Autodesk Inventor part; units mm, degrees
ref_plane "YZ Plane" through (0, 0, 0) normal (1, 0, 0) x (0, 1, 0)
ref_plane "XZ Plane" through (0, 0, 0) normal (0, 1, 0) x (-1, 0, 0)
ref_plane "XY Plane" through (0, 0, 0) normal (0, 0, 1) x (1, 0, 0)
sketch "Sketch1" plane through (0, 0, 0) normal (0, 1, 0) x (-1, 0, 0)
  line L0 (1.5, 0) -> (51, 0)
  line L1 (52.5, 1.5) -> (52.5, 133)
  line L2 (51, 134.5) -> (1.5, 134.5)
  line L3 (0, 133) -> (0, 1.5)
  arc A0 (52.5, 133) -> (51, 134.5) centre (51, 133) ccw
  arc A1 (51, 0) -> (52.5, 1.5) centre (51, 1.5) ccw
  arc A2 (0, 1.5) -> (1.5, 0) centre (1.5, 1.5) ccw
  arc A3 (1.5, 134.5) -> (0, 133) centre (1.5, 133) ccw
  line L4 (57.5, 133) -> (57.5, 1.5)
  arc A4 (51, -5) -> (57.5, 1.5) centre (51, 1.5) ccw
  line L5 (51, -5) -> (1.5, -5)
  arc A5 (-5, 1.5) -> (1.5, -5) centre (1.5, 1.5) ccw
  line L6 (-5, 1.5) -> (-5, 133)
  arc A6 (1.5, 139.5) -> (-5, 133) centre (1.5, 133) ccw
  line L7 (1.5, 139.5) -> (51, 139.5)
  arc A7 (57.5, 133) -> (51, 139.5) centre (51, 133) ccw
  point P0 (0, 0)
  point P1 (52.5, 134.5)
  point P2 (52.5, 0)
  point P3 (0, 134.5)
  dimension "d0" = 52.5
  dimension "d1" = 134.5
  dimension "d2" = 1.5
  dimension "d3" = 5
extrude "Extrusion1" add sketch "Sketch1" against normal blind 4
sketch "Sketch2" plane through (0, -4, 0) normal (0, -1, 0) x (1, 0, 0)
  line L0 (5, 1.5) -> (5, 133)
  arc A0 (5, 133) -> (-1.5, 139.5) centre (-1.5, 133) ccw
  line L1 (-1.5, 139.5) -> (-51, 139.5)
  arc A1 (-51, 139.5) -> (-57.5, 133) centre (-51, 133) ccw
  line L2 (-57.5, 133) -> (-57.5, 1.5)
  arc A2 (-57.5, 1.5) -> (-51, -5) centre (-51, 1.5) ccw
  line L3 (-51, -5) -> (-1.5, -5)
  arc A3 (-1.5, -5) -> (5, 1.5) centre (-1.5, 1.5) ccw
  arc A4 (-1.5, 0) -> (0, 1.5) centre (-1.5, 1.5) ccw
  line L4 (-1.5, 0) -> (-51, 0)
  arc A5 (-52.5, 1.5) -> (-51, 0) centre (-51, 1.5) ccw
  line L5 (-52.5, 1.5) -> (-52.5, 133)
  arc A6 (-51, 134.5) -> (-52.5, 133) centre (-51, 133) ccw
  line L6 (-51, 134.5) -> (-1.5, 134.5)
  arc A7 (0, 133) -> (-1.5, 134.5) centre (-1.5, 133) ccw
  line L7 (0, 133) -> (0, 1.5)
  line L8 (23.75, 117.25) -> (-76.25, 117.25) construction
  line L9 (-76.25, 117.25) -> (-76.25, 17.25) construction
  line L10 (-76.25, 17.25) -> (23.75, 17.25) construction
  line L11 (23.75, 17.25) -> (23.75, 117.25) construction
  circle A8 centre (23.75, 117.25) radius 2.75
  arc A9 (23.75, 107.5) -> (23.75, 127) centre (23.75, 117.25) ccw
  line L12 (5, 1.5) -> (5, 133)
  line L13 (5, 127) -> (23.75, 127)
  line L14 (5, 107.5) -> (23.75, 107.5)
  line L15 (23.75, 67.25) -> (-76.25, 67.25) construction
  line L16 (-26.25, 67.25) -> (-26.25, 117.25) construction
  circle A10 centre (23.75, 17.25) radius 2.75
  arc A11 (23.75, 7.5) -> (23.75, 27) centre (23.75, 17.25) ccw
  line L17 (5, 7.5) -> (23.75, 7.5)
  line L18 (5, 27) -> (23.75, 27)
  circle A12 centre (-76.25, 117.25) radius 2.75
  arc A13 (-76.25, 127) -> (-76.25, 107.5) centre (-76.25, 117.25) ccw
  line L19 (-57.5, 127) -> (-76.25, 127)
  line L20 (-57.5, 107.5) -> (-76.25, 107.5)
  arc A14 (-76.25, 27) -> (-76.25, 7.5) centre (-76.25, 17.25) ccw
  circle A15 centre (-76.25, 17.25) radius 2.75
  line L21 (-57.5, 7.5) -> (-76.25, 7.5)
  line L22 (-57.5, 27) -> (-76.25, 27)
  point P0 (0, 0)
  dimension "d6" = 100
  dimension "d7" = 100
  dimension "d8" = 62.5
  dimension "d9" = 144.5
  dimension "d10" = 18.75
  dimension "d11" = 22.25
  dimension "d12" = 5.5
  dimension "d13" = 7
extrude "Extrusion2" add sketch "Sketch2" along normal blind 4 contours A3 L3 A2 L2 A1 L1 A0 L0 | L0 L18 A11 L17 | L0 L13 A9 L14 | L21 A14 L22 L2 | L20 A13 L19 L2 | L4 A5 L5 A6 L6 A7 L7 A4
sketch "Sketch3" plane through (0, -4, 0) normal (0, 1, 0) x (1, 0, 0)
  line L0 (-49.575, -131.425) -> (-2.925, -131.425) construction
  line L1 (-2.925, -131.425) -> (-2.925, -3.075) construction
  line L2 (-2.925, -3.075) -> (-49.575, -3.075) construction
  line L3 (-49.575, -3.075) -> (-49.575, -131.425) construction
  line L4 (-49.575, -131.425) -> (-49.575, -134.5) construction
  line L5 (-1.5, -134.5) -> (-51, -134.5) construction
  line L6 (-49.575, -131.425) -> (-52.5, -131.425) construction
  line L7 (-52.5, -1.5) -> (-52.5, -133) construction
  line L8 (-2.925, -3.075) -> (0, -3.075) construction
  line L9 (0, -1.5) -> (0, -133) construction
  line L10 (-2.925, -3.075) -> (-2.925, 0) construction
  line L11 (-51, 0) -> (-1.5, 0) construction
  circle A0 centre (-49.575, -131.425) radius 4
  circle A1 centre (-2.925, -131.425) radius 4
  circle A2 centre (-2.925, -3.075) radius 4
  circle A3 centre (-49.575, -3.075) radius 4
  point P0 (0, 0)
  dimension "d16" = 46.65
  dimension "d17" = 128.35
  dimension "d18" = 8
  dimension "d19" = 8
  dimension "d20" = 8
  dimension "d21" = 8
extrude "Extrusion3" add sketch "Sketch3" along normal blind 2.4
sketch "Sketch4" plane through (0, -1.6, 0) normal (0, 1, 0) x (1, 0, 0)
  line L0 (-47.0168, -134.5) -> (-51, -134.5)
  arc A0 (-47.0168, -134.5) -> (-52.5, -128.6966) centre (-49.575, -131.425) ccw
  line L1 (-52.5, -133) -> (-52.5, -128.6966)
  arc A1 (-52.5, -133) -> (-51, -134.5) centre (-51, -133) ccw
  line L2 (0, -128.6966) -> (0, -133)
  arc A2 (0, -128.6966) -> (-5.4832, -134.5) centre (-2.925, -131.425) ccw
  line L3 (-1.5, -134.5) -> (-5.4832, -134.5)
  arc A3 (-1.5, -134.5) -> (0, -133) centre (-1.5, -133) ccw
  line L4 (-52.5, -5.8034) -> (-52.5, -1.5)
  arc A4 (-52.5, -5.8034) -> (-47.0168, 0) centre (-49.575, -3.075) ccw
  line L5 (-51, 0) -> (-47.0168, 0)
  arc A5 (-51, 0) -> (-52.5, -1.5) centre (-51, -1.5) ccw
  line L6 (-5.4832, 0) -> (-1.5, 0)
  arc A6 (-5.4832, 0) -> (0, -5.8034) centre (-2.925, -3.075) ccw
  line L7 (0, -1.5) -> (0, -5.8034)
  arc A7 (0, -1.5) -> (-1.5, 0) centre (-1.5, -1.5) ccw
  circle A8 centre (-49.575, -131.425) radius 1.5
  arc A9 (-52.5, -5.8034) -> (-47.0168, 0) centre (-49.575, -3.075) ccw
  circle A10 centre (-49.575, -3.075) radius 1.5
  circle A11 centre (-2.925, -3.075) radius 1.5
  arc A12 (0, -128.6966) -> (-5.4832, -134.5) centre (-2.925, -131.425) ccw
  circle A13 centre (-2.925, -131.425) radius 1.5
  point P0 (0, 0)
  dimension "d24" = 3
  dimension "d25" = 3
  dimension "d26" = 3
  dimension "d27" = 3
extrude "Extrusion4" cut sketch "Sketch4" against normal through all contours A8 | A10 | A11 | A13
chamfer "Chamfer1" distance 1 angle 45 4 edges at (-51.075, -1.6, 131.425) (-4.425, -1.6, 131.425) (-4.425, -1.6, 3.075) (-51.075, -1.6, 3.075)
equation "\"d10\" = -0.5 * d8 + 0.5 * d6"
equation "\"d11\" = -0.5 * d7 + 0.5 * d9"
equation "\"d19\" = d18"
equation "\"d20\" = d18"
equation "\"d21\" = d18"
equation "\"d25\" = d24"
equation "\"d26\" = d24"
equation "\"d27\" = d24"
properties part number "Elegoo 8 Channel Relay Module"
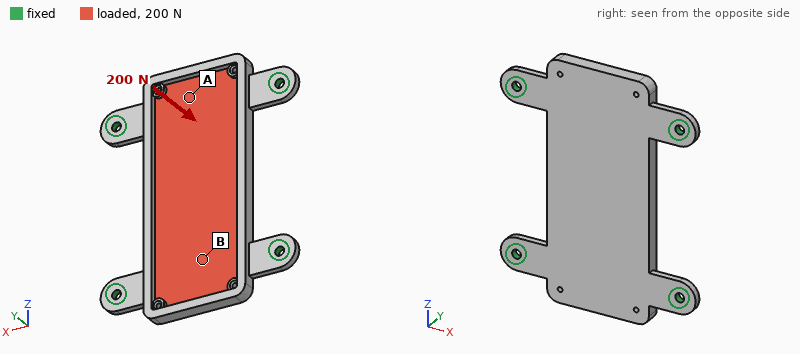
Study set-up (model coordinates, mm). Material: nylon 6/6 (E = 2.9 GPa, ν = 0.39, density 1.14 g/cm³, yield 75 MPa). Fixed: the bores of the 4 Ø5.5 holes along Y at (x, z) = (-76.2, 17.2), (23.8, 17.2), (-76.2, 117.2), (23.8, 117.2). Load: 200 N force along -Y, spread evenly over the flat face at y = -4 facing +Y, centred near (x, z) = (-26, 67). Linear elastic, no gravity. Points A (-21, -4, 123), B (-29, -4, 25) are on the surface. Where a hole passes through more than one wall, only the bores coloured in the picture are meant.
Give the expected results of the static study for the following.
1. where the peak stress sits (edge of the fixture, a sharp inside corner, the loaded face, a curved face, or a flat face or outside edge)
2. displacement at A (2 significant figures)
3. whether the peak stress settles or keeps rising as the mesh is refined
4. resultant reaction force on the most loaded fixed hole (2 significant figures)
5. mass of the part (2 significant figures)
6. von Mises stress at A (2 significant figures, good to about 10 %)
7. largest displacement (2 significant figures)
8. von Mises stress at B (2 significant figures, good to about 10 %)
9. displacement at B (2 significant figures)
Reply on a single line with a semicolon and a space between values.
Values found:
edge of the fixture; 0.40 mm; keeps rising; 52 N; 59 g; 2.9 MPa; 0.82 mm; 3.9 MPa; 0.54 mm
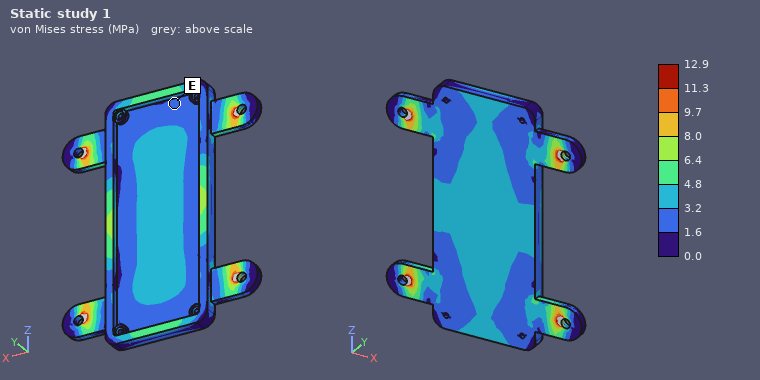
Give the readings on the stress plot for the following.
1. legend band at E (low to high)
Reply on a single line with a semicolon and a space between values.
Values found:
1.6 to 3.2 MPa
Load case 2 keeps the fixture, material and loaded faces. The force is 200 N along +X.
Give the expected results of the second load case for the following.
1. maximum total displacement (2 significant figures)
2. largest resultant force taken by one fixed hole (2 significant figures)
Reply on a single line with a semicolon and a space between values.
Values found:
36 µm; 51 N
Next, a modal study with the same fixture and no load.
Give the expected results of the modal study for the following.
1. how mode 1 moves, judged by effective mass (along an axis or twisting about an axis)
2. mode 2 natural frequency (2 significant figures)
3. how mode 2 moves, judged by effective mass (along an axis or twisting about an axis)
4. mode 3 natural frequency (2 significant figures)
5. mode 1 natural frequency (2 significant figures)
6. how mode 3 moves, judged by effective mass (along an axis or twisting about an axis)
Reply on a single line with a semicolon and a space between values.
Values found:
along Y; 620 Hz; twisting about X; 670 Hz; 450 Hz; along Y
